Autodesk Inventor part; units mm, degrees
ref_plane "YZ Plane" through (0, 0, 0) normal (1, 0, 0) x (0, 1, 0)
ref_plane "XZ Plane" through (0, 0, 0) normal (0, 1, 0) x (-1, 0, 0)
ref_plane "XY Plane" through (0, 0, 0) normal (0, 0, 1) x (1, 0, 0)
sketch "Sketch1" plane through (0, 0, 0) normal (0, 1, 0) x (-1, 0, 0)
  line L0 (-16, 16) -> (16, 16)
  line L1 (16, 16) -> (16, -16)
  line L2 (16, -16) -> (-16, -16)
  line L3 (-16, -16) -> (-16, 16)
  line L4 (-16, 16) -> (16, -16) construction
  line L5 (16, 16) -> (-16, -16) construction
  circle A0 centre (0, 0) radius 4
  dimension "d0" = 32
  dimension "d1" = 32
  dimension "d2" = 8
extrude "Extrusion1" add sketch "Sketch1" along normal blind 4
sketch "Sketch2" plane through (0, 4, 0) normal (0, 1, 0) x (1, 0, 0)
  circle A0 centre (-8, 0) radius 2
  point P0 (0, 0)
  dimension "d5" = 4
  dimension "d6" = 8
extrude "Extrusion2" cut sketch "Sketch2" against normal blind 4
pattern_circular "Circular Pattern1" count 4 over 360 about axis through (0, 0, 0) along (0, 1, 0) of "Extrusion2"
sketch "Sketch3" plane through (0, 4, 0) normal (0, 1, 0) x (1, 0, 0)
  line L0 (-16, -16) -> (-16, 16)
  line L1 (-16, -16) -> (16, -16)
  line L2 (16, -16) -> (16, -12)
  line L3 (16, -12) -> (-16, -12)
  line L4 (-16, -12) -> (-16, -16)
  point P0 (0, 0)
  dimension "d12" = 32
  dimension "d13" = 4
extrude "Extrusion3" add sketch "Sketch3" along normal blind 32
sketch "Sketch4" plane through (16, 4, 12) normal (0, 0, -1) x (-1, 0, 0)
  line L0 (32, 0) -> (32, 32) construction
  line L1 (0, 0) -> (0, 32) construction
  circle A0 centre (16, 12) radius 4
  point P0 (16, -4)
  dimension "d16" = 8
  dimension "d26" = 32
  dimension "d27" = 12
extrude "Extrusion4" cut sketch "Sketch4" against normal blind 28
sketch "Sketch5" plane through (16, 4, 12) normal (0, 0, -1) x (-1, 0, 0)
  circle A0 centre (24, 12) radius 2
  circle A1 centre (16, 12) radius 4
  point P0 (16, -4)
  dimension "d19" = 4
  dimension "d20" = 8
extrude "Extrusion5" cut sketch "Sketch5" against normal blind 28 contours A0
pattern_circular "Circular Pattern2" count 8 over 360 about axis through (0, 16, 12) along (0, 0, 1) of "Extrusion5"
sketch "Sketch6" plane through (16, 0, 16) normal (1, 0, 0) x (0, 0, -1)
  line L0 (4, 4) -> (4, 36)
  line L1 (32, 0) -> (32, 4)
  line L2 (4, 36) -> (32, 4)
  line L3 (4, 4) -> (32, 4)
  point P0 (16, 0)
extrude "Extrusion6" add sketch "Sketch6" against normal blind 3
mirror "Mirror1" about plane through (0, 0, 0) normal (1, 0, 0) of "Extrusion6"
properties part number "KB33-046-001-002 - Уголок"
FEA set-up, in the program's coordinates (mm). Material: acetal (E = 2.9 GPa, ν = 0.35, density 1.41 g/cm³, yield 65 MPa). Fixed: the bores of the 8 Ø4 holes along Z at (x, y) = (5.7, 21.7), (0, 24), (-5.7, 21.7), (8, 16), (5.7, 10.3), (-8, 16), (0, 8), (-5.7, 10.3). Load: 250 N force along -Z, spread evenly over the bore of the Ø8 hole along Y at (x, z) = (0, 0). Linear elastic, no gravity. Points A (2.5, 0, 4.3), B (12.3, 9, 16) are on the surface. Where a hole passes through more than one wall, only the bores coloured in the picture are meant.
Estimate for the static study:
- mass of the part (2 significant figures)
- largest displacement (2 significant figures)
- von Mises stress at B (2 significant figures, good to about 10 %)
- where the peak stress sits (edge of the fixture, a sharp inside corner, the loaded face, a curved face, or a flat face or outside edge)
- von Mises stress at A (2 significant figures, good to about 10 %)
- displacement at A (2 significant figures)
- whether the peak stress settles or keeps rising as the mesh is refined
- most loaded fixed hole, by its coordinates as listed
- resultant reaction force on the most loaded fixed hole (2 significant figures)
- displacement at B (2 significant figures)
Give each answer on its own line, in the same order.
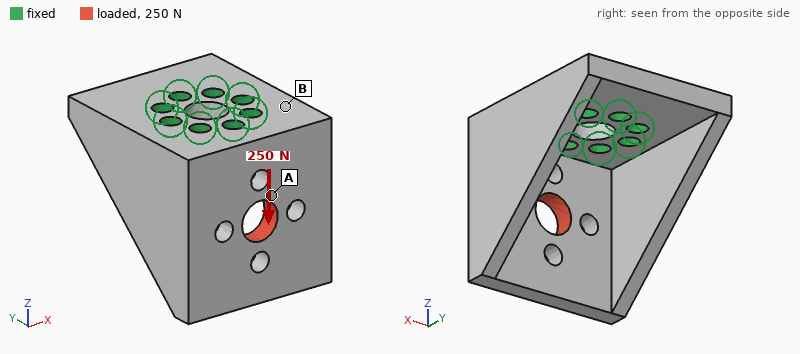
14 g
0.11 mm
2.2 MPa
edge of the fixture
5.6 MPa
0.072 mm
keeps rising
(0, 8)
120 N
0.018 mm
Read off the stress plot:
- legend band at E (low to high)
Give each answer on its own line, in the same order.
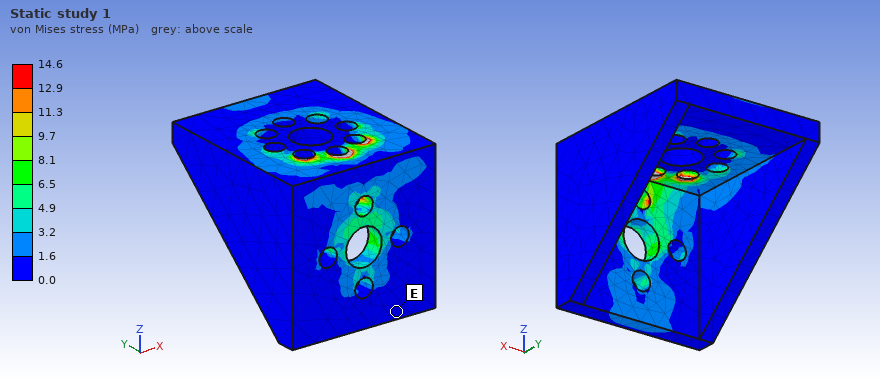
0.0 to 1.6 MPa
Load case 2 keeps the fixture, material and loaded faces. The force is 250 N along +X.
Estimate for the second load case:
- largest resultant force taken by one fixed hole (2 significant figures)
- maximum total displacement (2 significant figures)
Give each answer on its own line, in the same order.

140 N
0.34 mm
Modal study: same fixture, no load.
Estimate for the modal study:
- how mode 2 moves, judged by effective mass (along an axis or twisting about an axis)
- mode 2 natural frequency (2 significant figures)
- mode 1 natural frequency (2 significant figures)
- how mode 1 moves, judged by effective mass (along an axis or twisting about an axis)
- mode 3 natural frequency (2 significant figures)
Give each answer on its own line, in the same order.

along Y
2100 Hz
1700 Hz
along X
3600 Hz
